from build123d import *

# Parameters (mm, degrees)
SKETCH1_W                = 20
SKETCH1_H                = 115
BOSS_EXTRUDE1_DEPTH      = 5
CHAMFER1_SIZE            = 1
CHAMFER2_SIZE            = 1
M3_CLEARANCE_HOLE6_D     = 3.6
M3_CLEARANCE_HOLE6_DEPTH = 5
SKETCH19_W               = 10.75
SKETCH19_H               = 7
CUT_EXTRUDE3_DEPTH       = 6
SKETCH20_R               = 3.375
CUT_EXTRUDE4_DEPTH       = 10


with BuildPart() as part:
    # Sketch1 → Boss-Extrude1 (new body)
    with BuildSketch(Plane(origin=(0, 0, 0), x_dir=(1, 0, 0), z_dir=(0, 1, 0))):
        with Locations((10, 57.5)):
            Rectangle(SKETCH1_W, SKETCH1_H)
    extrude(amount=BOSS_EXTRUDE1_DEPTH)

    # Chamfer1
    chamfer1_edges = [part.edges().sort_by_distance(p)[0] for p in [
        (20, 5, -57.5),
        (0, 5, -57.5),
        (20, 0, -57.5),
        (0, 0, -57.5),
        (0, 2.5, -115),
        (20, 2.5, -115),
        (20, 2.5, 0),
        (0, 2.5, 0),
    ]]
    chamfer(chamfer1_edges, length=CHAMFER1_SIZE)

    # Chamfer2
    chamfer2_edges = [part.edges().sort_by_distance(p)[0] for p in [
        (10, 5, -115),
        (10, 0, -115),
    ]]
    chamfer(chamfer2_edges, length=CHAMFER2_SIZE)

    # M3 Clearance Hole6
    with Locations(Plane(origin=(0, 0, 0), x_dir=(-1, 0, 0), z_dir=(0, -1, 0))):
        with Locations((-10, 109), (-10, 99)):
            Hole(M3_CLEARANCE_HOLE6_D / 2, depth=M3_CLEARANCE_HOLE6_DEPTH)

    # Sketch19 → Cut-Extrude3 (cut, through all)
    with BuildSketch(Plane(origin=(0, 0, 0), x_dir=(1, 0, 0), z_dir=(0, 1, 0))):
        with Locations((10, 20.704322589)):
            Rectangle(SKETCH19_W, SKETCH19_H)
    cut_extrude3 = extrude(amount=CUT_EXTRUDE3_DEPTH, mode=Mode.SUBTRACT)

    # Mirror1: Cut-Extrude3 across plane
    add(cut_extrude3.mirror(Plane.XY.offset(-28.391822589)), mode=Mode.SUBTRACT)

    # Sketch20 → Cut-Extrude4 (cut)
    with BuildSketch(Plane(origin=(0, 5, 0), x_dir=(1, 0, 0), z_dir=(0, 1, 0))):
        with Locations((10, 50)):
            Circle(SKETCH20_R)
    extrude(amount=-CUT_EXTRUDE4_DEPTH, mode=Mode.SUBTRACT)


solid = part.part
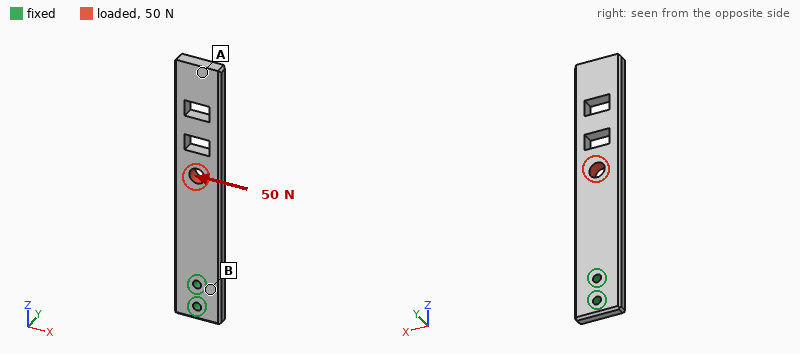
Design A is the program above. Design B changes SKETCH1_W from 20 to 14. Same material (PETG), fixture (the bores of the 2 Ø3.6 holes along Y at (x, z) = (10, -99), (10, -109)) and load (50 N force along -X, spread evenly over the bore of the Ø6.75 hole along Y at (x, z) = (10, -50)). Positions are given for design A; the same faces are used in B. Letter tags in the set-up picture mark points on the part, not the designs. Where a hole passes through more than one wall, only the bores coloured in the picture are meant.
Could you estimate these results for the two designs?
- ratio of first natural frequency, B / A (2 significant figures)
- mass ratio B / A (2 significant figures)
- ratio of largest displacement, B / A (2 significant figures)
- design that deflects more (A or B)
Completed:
1.00
0.66
2.4
B
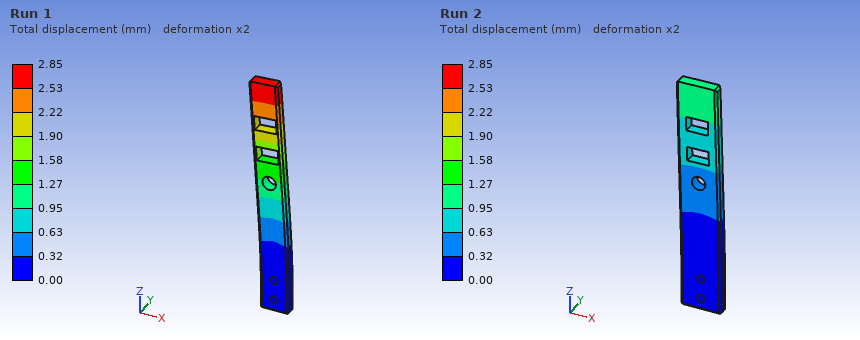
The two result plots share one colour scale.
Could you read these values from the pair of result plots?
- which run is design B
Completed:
Run 1
